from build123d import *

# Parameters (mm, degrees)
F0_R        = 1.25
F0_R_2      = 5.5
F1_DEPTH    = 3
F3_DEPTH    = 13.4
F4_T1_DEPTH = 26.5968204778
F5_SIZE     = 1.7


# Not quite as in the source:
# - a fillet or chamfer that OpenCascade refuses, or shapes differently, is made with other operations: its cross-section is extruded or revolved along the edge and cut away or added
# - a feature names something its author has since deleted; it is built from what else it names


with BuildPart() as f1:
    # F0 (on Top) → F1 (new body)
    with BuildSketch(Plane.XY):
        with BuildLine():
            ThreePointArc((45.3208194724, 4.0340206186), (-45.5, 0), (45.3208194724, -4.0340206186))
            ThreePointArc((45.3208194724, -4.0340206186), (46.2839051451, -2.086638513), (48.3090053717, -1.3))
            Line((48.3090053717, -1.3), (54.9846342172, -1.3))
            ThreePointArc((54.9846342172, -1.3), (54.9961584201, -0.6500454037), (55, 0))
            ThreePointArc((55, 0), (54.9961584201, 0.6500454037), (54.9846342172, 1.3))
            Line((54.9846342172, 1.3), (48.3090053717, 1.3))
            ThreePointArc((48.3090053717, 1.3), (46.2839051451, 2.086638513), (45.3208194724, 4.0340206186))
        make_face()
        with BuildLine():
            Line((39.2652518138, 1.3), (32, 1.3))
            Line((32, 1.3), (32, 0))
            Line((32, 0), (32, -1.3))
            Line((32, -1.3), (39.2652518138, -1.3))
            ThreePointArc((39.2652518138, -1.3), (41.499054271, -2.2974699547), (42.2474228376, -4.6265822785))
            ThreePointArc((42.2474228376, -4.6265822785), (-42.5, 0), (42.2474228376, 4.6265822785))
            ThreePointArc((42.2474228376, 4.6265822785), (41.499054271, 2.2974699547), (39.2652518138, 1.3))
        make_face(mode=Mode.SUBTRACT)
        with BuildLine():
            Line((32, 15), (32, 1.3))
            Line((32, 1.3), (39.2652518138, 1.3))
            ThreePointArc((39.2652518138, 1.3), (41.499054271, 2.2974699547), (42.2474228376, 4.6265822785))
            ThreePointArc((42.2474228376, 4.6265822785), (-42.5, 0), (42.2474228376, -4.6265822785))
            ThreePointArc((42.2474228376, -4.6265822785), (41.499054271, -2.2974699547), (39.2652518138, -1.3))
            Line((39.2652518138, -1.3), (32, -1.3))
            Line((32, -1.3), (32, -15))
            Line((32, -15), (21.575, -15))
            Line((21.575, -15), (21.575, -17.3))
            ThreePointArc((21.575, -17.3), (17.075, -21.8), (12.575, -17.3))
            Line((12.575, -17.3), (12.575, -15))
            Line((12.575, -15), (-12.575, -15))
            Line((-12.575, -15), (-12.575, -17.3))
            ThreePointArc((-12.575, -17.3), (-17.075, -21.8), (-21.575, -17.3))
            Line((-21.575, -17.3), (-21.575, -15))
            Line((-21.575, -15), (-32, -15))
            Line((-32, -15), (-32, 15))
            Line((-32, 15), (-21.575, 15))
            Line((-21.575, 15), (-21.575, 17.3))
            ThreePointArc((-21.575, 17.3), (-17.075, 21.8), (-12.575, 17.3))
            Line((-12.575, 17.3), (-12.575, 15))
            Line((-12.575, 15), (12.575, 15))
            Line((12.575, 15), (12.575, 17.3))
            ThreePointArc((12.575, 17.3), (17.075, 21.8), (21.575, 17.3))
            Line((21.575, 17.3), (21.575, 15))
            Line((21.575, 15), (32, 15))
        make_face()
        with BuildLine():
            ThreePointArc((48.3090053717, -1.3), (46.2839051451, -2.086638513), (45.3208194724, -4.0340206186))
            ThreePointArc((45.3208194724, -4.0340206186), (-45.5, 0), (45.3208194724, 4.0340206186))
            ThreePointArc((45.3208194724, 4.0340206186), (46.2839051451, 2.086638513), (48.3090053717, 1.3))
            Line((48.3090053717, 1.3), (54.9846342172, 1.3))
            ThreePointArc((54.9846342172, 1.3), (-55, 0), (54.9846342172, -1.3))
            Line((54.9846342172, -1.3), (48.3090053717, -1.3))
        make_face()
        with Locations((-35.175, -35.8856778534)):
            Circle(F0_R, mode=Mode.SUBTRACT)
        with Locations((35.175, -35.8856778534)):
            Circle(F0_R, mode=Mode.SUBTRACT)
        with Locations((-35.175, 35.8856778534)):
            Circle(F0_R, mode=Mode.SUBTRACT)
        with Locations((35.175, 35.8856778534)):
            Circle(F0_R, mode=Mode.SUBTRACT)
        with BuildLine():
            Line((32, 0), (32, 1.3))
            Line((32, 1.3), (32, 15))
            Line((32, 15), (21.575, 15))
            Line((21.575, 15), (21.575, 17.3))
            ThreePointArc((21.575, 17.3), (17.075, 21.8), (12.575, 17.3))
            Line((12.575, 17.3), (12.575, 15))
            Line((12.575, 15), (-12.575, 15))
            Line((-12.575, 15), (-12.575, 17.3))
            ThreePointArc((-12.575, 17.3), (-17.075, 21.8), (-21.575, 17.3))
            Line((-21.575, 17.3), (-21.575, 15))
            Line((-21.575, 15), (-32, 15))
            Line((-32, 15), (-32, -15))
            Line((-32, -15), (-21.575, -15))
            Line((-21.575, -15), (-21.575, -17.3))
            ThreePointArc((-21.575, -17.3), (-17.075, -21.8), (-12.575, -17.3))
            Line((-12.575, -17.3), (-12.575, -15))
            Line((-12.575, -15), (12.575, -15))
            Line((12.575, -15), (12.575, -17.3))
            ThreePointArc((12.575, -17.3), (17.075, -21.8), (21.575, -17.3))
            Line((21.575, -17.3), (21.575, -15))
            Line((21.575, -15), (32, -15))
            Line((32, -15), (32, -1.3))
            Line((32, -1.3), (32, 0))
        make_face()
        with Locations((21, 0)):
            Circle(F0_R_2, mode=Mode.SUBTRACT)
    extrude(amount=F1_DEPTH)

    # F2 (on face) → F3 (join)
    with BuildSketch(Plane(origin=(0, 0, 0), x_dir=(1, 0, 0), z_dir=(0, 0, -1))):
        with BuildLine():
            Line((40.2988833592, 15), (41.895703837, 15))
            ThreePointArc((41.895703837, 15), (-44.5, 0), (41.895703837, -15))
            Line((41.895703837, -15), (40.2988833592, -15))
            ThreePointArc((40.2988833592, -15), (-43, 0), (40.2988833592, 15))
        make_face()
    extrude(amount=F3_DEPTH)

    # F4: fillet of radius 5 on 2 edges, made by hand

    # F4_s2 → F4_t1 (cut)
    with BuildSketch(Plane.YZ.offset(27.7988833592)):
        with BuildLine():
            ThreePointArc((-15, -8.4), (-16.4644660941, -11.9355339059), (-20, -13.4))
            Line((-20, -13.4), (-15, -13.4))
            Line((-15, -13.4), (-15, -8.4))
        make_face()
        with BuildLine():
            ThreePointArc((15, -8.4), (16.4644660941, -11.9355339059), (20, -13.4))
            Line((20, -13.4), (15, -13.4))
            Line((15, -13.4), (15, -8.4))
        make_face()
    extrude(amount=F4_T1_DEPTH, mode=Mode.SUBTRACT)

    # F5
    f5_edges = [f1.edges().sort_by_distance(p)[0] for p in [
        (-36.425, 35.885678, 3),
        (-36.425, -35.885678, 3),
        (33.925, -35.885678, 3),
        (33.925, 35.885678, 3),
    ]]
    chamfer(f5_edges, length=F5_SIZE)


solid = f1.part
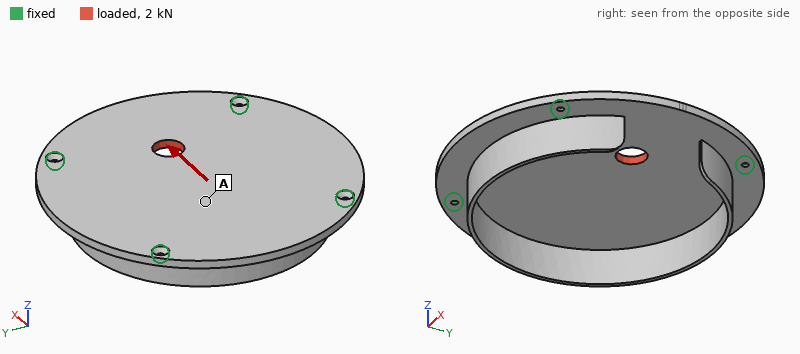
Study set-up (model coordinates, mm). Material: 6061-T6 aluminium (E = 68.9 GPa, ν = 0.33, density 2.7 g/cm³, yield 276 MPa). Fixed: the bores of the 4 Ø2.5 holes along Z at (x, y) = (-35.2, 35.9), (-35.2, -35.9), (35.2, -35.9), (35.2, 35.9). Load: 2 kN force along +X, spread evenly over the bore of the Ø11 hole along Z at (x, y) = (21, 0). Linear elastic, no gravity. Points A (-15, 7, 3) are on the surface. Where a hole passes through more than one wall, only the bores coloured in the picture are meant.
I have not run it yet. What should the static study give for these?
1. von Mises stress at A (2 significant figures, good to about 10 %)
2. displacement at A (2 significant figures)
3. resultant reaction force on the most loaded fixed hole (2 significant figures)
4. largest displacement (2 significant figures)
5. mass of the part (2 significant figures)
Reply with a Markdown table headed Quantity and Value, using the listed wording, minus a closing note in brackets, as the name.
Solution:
| Quantity | Value |
|---|---|
| von Mises stress at A | 4.9 MPa |
| displacement at A | 5.5 µm |
| resultant reaction force on the most loaded fixed hole | 550 N |
| largest displacement | 12 µm |
| mass of the part | 89 g |
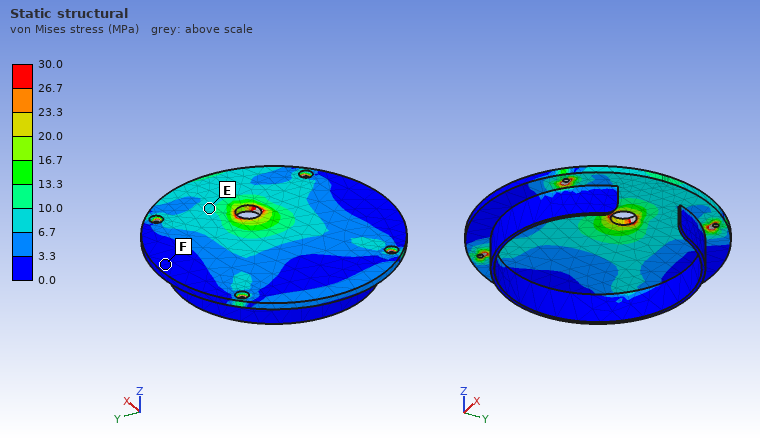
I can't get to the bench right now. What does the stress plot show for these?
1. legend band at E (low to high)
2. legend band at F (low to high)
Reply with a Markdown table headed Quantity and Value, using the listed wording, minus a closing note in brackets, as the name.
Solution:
| Quantity | Value |
|---|---|
| legend band at E | 6.7 to 10.0 MPa |
| legend band at F | 0.0 to 3.3 MPa |
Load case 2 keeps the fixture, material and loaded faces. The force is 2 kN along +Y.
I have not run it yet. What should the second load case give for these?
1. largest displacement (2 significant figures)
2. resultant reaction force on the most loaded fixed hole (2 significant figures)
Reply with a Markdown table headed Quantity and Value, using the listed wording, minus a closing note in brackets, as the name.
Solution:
| Quantity | Value |
|---|---|
| largest displacement | 9.6 µm |
| resultant reaction force on the most loaded fixed hole | 720 N |
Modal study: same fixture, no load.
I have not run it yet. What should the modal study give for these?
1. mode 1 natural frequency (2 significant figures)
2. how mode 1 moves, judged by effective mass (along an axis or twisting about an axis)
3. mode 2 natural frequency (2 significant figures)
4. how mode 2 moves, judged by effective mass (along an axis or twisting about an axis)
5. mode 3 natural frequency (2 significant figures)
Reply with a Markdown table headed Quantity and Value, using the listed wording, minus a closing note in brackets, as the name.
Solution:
| Quantity | Value |
|---|---|
| mode 1 natural frequency | 1900 Hz |
| how mode 1 moves, judged by effective mass | along Z |
| mode 2 natural frequency | 2300 Hz |
| how mode 2 moves, judged by effective mass | along Z |
| mode 3 natural frequency | 2800 Hz |
